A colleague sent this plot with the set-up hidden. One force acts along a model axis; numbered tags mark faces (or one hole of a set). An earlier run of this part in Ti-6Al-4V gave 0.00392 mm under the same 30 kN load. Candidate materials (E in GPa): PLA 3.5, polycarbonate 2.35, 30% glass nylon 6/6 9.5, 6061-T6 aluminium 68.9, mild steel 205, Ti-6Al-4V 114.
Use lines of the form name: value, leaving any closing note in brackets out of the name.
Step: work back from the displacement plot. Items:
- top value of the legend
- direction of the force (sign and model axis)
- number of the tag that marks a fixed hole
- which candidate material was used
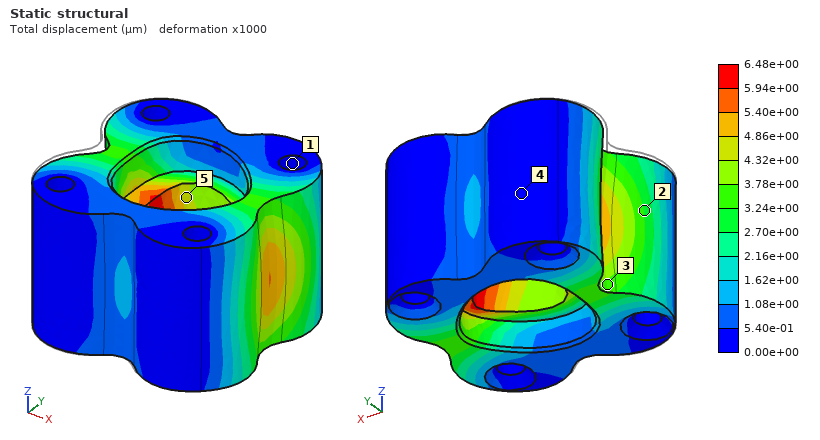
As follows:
top value of the legend: 6.48e+00 µm
direction of the force: +X
number of the tag that marks a fixed hole: 1
which candidate material was used: 6061-T6 aluminium
